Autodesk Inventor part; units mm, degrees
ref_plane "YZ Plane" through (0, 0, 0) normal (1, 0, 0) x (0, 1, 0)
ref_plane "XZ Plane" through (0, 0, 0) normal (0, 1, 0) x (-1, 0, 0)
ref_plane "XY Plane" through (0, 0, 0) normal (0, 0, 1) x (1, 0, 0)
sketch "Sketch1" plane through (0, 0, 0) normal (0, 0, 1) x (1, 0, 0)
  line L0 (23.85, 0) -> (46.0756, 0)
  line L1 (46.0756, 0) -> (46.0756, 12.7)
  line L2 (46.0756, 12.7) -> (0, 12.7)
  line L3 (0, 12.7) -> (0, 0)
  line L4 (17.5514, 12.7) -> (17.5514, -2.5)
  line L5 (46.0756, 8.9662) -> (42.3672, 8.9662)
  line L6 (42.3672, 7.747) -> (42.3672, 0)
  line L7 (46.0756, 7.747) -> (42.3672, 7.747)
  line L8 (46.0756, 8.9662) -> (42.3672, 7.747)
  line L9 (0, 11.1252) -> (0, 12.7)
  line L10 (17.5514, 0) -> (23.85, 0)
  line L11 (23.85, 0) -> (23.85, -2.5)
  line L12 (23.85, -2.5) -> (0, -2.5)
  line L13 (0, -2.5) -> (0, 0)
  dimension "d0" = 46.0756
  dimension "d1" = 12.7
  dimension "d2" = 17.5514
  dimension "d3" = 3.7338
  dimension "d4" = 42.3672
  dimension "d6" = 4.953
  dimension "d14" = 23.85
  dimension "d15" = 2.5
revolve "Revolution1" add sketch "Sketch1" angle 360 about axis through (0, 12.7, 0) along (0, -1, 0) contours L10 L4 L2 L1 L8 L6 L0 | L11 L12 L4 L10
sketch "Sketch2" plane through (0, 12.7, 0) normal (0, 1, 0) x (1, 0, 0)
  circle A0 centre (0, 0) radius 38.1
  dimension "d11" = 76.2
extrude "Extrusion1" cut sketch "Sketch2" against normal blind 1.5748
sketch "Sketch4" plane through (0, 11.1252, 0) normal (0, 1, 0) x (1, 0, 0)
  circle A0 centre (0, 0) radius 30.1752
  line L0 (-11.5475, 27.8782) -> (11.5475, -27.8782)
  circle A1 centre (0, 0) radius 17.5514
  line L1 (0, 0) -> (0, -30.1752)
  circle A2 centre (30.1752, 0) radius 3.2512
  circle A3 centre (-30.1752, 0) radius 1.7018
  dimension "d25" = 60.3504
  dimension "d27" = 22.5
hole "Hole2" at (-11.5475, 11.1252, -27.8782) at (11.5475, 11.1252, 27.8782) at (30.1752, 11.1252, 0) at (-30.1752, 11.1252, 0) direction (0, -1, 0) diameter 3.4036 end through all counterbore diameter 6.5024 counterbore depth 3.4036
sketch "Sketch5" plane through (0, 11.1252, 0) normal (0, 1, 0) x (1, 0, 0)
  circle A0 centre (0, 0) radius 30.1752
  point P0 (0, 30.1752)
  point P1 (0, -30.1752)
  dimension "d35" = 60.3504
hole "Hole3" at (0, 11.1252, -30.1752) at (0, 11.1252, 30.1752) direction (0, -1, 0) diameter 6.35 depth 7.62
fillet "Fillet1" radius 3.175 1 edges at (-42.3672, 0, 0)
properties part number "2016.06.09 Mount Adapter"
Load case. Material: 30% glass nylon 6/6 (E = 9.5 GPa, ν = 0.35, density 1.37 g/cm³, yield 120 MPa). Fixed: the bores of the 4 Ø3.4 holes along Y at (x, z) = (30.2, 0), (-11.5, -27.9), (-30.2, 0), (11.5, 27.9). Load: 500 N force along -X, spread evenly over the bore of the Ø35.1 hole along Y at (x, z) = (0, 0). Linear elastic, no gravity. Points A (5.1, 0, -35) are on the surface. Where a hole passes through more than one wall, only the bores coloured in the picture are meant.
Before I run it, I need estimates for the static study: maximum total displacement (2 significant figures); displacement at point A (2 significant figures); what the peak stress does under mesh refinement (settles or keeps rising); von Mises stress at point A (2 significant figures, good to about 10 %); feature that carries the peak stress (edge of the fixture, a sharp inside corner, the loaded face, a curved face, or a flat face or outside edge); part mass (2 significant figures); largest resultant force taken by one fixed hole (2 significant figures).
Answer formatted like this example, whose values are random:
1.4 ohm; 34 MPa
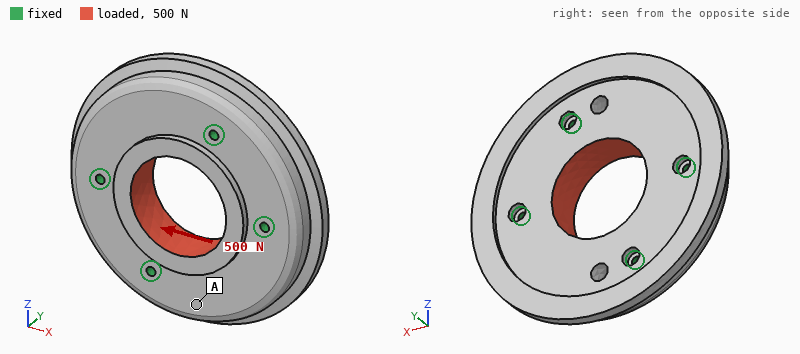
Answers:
2.0 µm; 0.78 µm; keeps rising; 0.27 MPa; edge of the fixture; 80 g; 130 N
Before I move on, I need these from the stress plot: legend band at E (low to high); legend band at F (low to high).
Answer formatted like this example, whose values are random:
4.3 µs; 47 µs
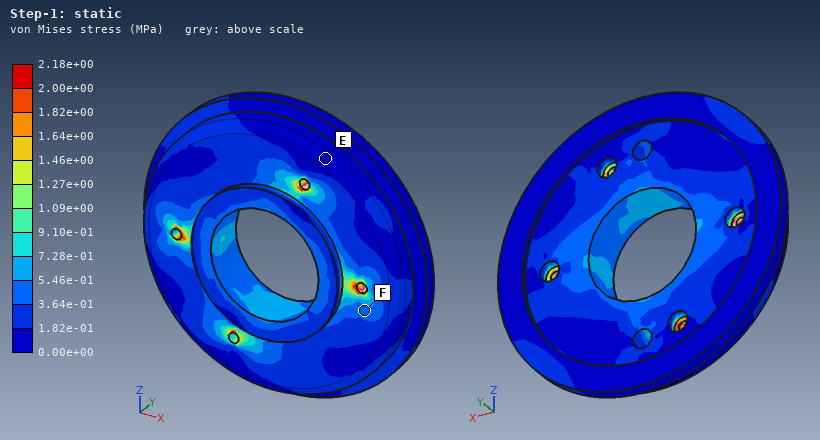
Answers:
0.00e+00 to 1.82e-01 MPa; 3.64e-01 to 5.46e-01 MPa
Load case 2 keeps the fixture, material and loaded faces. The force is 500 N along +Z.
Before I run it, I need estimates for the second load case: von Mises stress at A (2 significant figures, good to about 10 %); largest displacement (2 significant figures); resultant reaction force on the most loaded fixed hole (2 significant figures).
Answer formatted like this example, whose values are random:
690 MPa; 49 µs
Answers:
0.31 MPa; 2.5 µm; 130 N
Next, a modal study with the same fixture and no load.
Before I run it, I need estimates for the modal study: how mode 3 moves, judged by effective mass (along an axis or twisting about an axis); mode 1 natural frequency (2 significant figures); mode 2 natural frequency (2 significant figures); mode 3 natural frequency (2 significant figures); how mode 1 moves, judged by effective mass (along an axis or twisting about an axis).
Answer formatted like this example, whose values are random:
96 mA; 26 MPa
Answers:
along Y; 3800 Hz; 4200 Hz; 7600 Hz; along Y
